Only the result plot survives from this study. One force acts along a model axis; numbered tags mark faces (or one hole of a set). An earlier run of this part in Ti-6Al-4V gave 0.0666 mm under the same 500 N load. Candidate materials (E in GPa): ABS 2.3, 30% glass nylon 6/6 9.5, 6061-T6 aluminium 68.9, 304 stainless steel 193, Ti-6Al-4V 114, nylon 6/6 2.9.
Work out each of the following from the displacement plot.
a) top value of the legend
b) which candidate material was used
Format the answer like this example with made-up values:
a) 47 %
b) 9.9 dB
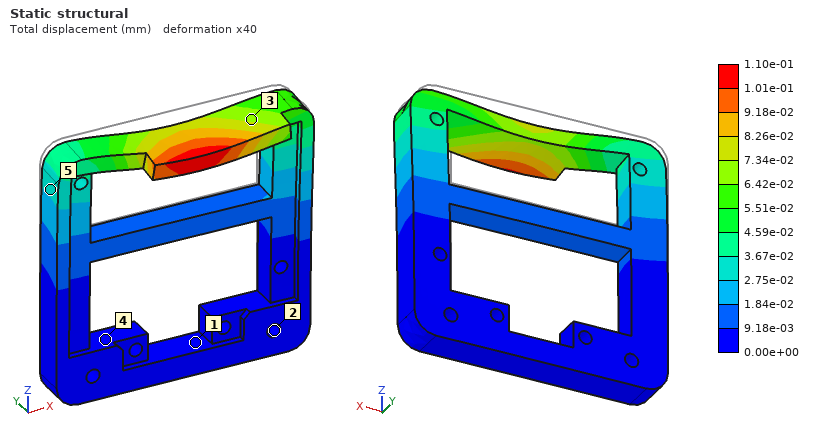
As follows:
a) 1.10e-01 mm
b) 6061-T6 aluminium
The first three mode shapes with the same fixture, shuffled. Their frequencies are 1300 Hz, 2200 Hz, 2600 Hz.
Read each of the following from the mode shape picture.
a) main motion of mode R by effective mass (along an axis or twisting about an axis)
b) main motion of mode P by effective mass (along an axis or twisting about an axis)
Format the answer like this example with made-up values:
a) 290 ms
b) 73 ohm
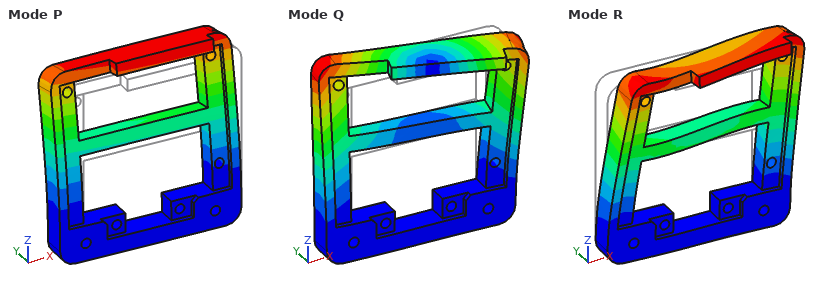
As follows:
a) along X
b) along Y
